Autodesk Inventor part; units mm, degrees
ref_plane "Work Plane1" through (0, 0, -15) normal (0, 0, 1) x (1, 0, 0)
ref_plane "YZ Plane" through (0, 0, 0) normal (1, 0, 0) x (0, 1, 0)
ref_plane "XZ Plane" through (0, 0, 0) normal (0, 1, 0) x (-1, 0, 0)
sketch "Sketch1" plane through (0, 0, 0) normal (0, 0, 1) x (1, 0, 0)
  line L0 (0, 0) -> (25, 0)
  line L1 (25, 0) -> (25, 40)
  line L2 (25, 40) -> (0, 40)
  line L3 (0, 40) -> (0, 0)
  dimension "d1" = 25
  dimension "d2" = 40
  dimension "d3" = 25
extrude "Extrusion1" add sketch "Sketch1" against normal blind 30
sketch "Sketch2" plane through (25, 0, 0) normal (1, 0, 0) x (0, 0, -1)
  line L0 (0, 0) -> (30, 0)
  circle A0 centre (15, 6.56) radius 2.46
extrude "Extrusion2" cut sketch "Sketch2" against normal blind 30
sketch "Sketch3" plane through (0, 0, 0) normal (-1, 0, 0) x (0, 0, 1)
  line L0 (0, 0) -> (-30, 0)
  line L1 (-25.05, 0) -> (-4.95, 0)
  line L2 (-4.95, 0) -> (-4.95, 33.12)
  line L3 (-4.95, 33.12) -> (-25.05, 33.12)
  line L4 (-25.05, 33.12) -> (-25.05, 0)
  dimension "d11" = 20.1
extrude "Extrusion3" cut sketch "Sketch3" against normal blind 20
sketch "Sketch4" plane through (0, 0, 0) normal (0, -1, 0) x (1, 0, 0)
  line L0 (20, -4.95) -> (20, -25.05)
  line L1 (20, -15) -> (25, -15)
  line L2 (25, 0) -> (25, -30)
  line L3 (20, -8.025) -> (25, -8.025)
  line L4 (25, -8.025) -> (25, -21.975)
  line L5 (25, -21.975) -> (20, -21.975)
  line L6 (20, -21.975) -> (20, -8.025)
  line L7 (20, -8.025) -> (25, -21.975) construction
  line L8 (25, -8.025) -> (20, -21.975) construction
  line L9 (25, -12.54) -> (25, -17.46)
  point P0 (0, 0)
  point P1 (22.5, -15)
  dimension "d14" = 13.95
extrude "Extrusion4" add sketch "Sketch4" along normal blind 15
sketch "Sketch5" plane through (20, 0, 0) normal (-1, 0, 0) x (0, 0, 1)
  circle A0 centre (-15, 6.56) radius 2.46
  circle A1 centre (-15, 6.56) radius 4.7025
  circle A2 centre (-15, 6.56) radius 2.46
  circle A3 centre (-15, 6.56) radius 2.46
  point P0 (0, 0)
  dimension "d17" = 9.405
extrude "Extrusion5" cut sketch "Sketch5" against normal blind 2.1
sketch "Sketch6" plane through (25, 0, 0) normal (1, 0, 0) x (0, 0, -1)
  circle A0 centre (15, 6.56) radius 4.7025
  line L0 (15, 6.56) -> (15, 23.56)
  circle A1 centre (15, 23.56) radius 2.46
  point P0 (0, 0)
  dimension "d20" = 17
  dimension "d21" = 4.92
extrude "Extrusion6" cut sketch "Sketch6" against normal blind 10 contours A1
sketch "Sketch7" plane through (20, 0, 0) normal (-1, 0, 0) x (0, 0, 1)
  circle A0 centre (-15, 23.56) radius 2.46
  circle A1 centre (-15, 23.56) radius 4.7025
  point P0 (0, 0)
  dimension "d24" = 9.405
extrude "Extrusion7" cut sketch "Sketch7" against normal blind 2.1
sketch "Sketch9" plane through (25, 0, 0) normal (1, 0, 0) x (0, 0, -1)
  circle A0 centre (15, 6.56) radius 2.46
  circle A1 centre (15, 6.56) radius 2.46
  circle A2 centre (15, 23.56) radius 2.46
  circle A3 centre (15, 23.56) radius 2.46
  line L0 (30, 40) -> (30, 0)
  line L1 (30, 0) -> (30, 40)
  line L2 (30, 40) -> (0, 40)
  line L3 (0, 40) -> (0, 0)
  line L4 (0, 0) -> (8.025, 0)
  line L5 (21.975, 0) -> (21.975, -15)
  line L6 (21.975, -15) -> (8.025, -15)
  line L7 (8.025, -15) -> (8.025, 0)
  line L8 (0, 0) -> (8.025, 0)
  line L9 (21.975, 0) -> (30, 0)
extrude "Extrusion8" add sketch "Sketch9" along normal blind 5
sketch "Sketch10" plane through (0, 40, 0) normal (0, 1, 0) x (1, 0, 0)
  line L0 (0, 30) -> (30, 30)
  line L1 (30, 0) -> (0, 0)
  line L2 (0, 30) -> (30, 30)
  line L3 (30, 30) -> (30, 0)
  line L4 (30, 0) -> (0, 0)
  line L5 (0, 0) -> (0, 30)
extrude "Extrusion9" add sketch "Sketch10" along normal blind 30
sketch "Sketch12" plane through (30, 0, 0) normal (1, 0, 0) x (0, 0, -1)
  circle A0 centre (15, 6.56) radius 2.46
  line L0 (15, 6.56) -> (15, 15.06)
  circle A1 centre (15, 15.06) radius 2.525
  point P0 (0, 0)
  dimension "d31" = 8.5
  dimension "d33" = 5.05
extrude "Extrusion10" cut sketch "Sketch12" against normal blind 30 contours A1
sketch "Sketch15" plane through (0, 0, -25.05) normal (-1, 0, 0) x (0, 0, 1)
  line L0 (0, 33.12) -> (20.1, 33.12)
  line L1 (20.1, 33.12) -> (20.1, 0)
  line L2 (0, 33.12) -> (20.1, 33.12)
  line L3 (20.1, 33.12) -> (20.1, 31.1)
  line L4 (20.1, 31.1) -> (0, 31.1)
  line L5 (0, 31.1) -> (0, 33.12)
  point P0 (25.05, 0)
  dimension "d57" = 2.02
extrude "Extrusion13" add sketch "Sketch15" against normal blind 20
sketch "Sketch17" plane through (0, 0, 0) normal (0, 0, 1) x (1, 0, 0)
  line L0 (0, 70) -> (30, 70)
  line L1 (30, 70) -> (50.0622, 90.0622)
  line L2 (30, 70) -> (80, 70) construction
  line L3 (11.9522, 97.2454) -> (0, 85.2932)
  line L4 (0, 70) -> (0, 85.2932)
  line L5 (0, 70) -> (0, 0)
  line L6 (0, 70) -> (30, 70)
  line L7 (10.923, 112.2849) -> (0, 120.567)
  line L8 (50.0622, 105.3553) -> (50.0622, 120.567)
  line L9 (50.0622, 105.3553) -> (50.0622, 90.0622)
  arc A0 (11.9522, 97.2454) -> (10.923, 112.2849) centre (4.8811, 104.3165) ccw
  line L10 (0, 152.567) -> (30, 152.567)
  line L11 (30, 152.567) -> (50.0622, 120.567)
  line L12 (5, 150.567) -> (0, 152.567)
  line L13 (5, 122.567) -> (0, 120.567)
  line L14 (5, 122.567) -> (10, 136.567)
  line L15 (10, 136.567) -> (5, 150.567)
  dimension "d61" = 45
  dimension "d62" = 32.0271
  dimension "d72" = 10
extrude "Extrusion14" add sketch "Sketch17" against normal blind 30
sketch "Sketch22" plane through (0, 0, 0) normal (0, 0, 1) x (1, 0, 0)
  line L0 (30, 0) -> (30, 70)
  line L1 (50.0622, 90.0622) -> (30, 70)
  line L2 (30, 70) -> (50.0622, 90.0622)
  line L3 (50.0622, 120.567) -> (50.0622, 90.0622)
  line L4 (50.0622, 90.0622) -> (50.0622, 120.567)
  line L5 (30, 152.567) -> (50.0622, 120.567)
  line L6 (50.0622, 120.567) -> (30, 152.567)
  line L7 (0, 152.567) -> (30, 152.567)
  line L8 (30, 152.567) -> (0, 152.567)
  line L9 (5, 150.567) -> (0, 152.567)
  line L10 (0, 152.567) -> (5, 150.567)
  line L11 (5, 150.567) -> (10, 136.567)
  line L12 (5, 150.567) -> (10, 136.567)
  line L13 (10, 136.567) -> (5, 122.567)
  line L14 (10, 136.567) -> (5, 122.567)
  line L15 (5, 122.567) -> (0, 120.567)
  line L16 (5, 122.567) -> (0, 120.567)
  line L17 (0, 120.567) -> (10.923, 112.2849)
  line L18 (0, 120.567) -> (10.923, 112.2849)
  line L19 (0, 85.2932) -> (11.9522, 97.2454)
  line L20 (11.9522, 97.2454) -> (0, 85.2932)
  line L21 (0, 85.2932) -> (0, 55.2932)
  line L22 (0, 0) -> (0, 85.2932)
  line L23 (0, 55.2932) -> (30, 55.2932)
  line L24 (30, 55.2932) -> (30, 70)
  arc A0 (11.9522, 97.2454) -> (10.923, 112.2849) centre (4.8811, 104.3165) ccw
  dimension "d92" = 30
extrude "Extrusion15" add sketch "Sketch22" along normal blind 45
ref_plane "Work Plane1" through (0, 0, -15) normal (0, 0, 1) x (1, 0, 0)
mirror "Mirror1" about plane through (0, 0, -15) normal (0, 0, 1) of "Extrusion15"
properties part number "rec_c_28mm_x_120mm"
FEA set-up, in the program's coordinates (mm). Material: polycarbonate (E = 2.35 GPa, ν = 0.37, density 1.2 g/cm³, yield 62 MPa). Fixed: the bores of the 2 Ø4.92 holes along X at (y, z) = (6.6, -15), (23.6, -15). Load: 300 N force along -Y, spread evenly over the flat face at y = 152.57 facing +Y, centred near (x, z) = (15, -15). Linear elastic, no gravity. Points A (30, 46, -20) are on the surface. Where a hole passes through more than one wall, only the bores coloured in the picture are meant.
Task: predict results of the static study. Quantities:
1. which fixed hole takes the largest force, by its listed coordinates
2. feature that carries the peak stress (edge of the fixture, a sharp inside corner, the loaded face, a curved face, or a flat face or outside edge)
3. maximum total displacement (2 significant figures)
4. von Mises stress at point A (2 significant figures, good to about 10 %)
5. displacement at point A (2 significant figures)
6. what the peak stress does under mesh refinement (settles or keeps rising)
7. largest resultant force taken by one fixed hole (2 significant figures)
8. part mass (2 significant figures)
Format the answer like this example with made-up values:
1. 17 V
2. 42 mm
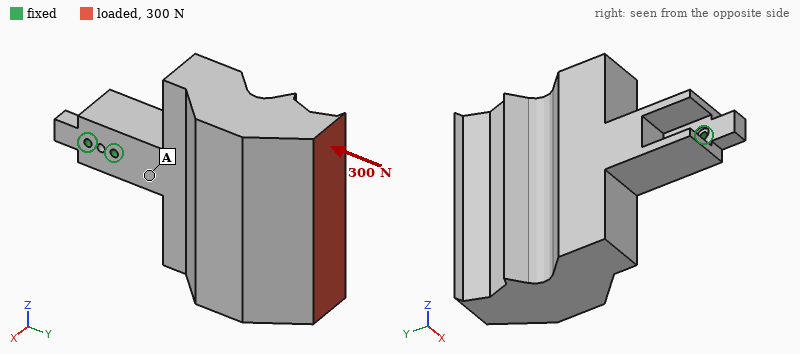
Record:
1. (23.6, -15)
2. edge of the fixture
3. 0.29 mm
4. 0.37 MPa
5. 0.046 mm
6. keeps rising
7. 230 N
8. 550 g
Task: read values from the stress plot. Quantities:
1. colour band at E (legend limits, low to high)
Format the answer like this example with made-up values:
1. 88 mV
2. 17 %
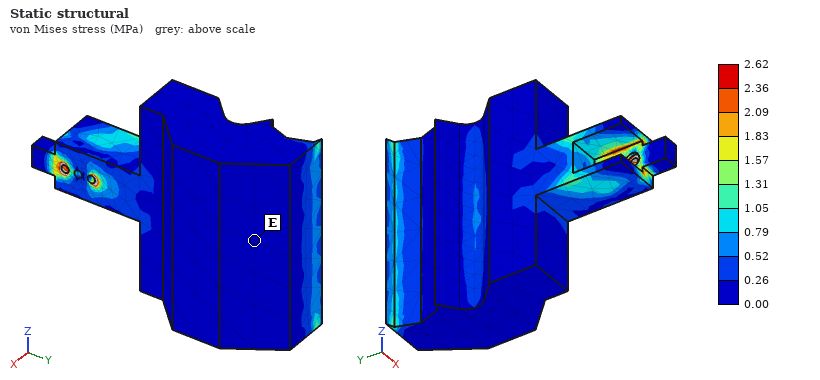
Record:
1. 0.00 to 0.26 MPa
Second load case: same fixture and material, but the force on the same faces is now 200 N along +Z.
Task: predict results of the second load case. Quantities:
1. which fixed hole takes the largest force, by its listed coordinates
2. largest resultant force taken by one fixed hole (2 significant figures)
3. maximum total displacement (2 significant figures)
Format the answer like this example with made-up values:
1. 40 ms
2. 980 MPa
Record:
1. (23.6, -15)
2. 1.3 kN
3. 2.3 mm
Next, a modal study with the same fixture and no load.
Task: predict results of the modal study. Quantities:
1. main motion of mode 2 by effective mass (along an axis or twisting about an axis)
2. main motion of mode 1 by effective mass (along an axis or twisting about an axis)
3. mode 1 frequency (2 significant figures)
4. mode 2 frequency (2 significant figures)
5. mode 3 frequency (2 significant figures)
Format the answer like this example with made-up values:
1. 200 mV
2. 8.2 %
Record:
1. along Z
2. along X
3. 93 Hz
4. 99 Hz
5. 150 Hz
